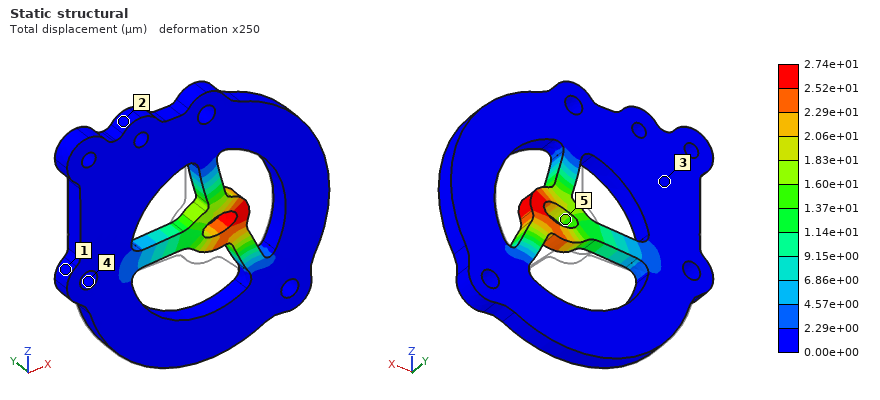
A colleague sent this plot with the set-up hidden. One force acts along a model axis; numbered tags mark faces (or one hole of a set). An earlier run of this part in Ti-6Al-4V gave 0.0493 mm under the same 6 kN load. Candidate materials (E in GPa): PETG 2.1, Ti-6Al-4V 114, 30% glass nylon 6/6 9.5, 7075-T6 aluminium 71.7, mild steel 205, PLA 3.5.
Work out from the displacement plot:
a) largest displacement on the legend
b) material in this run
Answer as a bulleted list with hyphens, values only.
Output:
- 2.74e+01 µm
- mild steel
